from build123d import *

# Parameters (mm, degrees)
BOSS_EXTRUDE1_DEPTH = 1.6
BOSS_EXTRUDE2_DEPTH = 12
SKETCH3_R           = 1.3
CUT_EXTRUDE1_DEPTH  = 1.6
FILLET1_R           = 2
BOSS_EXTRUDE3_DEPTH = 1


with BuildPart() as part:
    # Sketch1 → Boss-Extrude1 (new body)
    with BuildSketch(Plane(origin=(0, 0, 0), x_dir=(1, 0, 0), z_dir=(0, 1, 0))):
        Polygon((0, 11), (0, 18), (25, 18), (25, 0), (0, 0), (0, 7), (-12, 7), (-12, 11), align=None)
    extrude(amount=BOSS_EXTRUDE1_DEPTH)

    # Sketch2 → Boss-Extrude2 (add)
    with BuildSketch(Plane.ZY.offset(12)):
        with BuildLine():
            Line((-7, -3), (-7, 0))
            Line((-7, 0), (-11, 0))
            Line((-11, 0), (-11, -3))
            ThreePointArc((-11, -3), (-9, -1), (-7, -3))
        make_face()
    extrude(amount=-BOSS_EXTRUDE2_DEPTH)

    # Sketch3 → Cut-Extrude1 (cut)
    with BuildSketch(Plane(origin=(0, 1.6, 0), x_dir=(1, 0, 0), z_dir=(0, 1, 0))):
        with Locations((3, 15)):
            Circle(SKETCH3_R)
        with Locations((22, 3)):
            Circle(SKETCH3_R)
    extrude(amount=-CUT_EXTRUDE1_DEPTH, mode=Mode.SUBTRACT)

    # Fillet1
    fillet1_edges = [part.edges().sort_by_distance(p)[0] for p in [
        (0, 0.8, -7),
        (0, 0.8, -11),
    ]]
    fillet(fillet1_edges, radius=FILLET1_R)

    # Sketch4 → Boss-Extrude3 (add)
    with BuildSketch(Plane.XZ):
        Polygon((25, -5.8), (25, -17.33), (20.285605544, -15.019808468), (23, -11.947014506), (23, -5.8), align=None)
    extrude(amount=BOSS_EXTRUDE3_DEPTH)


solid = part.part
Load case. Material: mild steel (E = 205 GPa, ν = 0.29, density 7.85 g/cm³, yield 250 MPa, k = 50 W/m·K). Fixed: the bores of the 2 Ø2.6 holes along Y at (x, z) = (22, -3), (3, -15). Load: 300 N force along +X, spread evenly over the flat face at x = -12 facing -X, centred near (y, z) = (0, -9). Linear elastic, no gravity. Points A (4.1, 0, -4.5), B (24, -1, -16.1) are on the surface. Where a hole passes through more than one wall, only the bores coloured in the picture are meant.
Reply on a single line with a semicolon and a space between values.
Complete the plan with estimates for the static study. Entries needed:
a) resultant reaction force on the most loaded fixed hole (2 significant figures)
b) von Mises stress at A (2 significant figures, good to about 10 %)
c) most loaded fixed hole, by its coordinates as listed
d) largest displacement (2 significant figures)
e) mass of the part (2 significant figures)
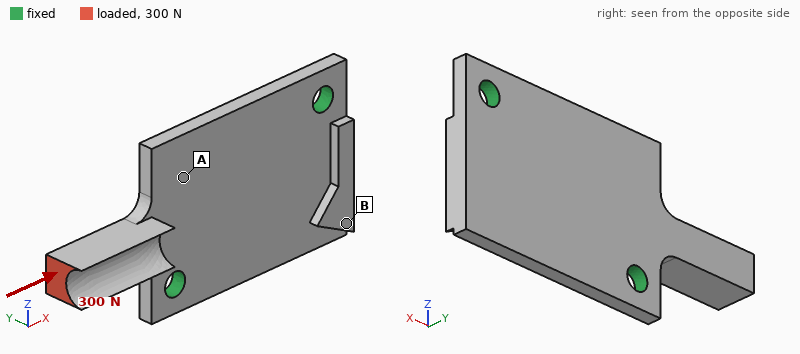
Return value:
180 N; 30 MPa; (3, -15); 32 µm; 6.9 g
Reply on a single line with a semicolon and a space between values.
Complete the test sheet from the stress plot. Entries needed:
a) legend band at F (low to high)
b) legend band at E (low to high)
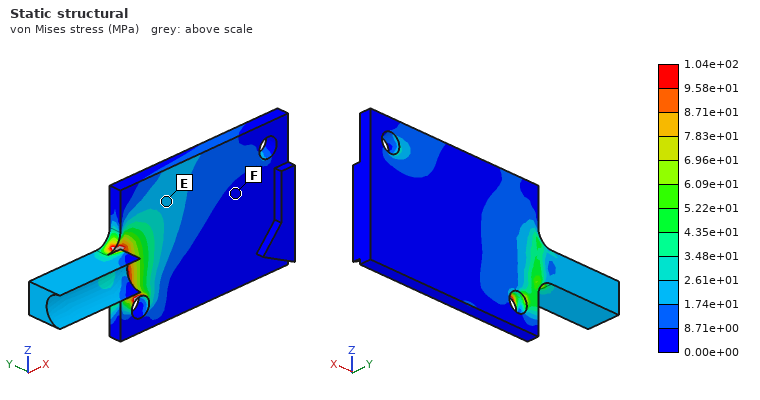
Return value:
0.00e+00 to 8.71e+00 MPa; 1.74e+01 to 2.61e+01 MPa
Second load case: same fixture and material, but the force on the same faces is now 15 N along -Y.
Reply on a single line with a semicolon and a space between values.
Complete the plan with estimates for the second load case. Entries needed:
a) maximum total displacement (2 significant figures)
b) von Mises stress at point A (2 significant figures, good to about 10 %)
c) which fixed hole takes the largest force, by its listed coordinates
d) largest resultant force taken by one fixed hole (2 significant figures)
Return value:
34 µm; 18 MPa; (3, -15); 20 N
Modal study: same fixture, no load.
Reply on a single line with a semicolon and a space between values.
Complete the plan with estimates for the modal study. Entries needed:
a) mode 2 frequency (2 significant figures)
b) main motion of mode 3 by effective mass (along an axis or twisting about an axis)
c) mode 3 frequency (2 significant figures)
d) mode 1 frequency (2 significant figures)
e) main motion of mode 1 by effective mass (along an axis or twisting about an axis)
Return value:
7900 Hz; along Y; 9700 Hz; 5100 Hz; along Y
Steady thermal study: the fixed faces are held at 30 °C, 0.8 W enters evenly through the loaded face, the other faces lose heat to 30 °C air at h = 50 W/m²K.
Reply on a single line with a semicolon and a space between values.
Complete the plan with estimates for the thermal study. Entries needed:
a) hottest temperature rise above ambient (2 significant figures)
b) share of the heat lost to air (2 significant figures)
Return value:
20 K; 27 %
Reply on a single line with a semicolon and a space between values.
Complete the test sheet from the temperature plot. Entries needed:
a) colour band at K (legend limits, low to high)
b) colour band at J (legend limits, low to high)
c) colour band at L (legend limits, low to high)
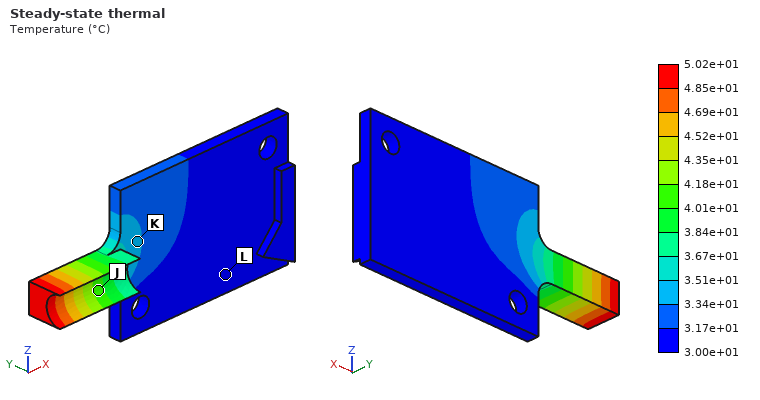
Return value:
3.34e+01 to 3.51e+01 °C; 4.01e+01 to 4.18e+01 °C; 3.00e+01 to 3.17e+01 °C
